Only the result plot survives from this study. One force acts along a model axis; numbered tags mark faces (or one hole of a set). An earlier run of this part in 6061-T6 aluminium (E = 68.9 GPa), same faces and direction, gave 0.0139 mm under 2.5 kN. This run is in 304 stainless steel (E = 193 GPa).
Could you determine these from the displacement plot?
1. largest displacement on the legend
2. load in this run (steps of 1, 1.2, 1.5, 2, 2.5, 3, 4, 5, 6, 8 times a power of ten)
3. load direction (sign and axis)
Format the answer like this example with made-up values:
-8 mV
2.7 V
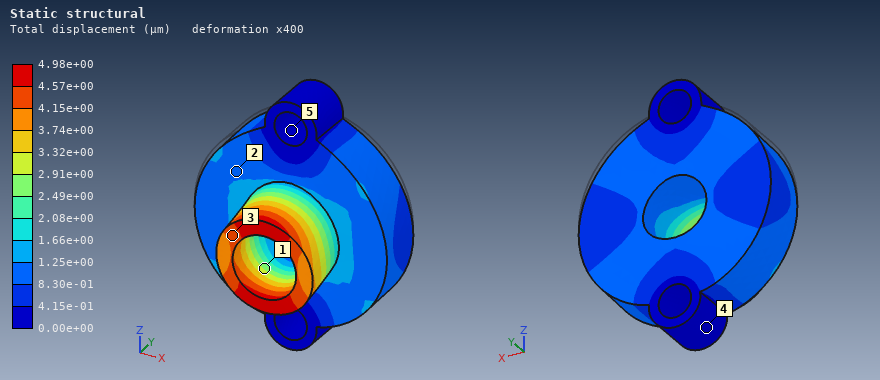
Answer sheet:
4.98e+00 µm
2.5 kN
-Z
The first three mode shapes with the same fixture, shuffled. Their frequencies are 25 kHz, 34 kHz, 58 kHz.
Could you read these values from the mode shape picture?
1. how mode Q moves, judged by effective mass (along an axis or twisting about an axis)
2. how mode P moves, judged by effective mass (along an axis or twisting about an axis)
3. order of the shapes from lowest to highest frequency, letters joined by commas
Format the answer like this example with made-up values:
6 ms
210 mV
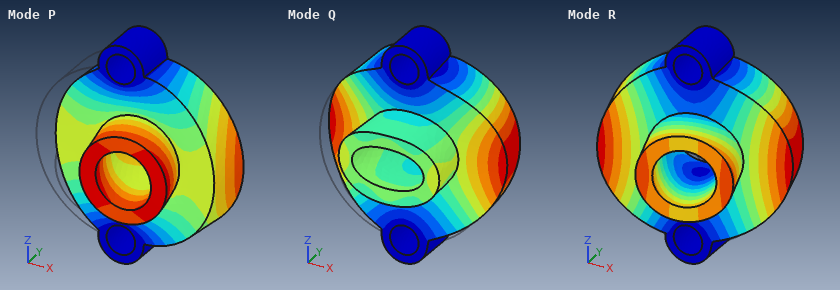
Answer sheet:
along Y
along X
R, Q, P
